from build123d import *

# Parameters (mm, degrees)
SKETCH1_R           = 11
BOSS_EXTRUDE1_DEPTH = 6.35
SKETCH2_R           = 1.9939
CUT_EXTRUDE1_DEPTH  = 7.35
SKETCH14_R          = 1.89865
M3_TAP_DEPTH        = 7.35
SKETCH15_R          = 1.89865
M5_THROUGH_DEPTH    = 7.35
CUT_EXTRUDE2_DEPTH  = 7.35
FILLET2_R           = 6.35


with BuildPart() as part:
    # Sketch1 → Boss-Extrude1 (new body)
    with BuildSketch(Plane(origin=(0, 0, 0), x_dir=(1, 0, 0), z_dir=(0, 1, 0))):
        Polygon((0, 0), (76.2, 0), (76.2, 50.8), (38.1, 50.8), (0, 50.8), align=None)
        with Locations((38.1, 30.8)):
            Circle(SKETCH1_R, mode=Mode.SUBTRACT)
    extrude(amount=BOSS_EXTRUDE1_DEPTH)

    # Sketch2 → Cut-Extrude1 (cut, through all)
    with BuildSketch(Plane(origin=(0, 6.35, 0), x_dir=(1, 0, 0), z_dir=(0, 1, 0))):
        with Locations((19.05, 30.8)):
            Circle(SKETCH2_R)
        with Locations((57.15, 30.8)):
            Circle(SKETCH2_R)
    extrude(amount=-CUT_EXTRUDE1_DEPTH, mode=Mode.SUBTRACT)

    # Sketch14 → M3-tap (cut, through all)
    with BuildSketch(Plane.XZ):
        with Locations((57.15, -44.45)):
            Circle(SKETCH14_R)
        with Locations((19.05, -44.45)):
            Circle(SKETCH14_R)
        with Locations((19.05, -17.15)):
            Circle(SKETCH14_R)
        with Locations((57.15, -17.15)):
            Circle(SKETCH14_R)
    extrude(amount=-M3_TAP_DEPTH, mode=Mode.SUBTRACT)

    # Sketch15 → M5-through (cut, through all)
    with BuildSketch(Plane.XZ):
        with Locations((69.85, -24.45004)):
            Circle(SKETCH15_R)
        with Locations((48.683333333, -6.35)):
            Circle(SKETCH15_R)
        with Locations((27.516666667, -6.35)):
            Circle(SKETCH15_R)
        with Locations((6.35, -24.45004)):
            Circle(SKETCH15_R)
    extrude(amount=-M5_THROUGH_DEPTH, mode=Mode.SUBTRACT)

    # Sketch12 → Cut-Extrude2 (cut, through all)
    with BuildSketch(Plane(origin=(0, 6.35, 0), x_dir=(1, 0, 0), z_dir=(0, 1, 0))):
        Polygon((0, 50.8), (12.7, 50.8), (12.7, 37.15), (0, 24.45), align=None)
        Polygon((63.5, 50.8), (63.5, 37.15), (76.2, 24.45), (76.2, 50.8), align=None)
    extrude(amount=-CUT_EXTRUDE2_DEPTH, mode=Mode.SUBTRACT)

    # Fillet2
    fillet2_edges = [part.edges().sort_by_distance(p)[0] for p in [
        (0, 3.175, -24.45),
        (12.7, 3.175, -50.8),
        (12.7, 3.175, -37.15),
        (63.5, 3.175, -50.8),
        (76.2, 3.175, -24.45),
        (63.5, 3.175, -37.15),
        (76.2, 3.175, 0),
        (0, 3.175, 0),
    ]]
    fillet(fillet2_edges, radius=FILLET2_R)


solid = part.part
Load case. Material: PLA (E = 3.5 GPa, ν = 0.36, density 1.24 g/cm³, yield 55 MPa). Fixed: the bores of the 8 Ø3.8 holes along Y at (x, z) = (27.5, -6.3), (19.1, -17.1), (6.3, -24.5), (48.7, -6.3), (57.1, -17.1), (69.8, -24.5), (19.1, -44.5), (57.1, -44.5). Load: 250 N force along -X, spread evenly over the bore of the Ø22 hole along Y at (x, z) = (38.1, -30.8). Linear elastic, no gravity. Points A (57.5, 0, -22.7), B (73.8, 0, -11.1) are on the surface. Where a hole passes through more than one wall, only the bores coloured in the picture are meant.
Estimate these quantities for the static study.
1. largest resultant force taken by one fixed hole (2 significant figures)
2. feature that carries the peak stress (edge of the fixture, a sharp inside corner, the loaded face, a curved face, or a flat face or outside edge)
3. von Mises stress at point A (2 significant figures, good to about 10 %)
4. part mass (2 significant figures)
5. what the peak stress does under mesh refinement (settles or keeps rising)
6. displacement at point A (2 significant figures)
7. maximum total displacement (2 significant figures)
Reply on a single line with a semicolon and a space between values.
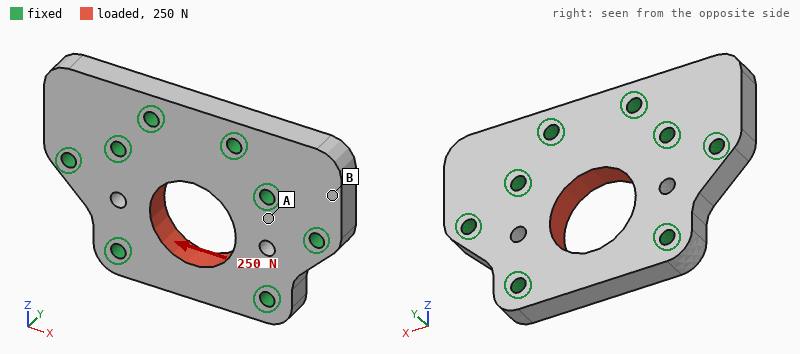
56 N; edge of the fixture; 0.43 MPa; 22 g; keeps rising; 1.0 µm; 3.3 µm
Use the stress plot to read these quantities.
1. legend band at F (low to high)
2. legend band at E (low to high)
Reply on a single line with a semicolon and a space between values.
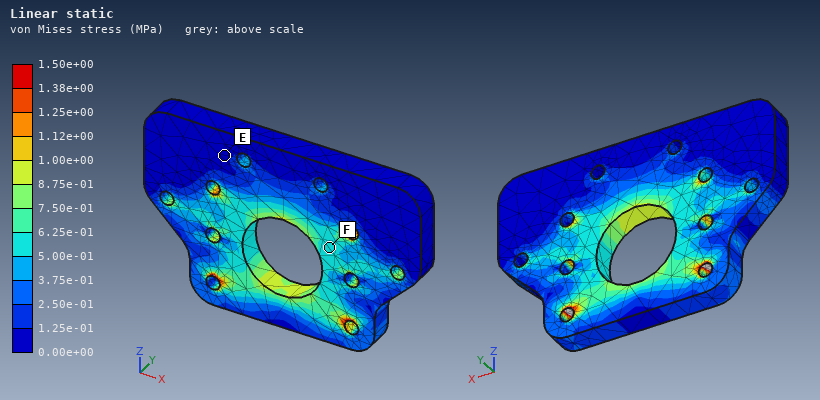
5.00e-01 to 6.25e-01 MPa; 0.00e+00 to 1.25e-01 MPa
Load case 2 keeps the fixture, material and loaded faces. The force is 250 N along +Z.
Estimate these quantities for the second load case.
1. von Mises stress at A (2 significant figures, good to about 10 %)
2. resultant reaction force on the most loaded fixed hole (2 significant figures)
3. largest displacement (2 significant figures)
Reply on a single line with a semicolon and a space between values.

0.46 MPa; 48 N; 9.9 µm
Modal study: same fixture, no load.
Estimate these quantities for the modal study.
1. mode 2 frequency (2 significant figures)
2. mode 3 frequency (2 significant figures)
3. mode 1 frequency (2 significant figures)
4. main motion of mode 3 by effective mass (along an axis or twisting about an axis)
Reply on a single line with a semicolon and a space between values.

5300 Hz; 7200 Hz; 5300 Hz; along Y
